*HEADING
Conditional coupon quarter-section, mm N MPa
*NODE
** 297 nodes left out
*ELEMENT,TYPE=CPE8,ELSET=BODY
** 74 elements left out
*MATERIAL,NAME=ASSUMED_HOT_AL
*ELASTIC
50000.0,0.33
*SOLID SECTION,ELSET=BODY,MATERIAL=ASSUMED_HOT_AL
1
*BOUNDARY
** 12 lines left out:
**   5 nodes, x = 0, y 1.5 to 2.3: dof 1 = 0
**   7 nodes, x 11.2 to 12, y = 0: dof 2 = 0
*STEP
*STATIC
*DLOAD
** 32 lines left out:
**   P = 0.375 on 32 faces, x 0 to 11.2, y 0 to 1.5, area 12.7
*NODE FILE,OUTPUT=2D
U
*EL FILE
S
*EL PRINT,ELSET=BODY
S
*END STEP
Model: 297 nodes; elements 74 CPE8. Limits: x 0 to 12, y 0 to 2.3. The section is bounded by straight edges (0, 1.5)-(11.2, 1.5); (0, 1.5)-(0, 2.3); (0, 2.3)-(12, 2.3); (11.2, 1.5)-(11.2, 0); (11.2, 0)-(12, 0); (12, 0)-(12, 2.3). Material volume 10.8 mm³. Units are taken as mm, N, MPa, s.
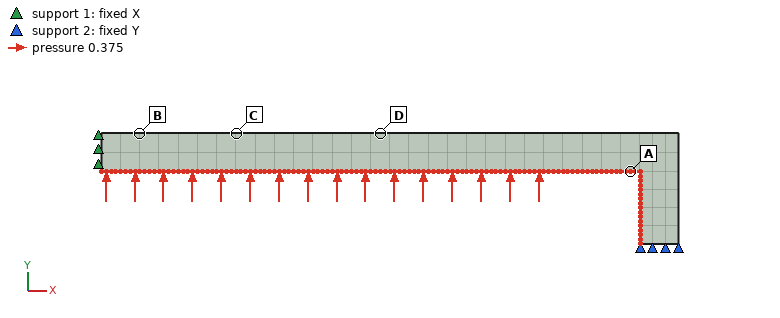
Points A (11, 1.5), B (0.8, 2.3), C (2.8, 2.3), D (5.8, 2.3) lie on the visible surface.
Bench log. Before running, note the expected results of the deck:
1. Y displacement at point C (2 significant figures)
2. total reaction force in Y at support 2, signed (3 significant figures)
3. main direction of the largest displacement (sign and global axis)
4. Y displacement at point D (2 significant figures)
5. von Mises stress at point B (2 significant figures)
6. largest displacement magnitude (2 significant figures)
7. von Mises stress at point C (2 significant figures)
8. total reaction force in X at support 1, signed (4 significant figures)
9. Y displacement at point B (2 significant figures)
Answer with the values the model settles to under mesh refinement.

0.16 mm
-4.20 N
+Y
0.11 mm
86 MPa
0.18 mm
75 MPa
-0.5625 N
0.18 mm
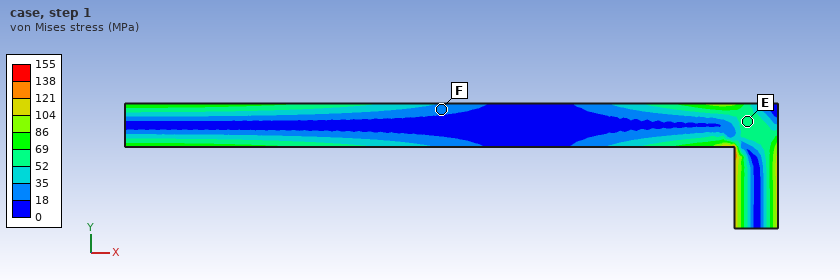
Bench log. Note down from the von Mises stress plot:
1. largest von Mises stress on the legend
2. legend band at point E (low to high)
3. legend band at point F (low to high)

155 MPa
52 to 69 MPa
18 to 35 MPa
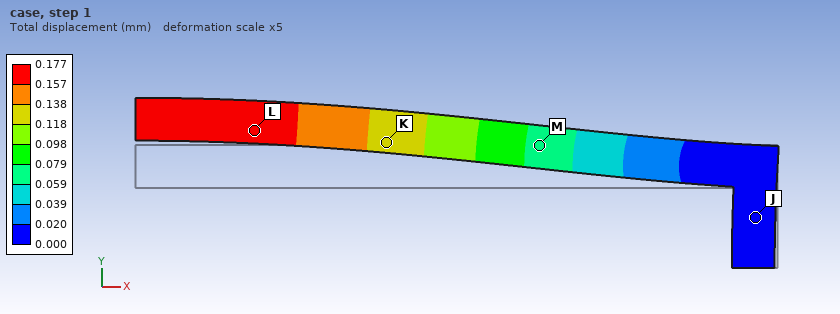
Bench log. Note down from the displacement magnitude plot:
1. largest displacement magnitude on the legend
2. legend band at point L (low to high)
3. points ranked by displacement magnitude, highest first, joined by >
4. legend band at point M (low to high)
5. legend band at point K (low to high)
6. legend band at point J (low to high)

0.177 mm
0.157 to 0.177 mm
L > K > M > J
0.059 to 0.079 mm
0.118 to 0.138 mm
0.000 to 0.020 mm
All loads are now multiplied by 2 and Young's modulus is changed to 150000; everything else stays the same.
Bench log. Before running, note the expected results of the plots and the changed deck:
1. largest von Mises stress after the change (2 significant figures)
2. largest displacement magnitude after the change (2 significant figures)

310 MPa
0.12 mm
